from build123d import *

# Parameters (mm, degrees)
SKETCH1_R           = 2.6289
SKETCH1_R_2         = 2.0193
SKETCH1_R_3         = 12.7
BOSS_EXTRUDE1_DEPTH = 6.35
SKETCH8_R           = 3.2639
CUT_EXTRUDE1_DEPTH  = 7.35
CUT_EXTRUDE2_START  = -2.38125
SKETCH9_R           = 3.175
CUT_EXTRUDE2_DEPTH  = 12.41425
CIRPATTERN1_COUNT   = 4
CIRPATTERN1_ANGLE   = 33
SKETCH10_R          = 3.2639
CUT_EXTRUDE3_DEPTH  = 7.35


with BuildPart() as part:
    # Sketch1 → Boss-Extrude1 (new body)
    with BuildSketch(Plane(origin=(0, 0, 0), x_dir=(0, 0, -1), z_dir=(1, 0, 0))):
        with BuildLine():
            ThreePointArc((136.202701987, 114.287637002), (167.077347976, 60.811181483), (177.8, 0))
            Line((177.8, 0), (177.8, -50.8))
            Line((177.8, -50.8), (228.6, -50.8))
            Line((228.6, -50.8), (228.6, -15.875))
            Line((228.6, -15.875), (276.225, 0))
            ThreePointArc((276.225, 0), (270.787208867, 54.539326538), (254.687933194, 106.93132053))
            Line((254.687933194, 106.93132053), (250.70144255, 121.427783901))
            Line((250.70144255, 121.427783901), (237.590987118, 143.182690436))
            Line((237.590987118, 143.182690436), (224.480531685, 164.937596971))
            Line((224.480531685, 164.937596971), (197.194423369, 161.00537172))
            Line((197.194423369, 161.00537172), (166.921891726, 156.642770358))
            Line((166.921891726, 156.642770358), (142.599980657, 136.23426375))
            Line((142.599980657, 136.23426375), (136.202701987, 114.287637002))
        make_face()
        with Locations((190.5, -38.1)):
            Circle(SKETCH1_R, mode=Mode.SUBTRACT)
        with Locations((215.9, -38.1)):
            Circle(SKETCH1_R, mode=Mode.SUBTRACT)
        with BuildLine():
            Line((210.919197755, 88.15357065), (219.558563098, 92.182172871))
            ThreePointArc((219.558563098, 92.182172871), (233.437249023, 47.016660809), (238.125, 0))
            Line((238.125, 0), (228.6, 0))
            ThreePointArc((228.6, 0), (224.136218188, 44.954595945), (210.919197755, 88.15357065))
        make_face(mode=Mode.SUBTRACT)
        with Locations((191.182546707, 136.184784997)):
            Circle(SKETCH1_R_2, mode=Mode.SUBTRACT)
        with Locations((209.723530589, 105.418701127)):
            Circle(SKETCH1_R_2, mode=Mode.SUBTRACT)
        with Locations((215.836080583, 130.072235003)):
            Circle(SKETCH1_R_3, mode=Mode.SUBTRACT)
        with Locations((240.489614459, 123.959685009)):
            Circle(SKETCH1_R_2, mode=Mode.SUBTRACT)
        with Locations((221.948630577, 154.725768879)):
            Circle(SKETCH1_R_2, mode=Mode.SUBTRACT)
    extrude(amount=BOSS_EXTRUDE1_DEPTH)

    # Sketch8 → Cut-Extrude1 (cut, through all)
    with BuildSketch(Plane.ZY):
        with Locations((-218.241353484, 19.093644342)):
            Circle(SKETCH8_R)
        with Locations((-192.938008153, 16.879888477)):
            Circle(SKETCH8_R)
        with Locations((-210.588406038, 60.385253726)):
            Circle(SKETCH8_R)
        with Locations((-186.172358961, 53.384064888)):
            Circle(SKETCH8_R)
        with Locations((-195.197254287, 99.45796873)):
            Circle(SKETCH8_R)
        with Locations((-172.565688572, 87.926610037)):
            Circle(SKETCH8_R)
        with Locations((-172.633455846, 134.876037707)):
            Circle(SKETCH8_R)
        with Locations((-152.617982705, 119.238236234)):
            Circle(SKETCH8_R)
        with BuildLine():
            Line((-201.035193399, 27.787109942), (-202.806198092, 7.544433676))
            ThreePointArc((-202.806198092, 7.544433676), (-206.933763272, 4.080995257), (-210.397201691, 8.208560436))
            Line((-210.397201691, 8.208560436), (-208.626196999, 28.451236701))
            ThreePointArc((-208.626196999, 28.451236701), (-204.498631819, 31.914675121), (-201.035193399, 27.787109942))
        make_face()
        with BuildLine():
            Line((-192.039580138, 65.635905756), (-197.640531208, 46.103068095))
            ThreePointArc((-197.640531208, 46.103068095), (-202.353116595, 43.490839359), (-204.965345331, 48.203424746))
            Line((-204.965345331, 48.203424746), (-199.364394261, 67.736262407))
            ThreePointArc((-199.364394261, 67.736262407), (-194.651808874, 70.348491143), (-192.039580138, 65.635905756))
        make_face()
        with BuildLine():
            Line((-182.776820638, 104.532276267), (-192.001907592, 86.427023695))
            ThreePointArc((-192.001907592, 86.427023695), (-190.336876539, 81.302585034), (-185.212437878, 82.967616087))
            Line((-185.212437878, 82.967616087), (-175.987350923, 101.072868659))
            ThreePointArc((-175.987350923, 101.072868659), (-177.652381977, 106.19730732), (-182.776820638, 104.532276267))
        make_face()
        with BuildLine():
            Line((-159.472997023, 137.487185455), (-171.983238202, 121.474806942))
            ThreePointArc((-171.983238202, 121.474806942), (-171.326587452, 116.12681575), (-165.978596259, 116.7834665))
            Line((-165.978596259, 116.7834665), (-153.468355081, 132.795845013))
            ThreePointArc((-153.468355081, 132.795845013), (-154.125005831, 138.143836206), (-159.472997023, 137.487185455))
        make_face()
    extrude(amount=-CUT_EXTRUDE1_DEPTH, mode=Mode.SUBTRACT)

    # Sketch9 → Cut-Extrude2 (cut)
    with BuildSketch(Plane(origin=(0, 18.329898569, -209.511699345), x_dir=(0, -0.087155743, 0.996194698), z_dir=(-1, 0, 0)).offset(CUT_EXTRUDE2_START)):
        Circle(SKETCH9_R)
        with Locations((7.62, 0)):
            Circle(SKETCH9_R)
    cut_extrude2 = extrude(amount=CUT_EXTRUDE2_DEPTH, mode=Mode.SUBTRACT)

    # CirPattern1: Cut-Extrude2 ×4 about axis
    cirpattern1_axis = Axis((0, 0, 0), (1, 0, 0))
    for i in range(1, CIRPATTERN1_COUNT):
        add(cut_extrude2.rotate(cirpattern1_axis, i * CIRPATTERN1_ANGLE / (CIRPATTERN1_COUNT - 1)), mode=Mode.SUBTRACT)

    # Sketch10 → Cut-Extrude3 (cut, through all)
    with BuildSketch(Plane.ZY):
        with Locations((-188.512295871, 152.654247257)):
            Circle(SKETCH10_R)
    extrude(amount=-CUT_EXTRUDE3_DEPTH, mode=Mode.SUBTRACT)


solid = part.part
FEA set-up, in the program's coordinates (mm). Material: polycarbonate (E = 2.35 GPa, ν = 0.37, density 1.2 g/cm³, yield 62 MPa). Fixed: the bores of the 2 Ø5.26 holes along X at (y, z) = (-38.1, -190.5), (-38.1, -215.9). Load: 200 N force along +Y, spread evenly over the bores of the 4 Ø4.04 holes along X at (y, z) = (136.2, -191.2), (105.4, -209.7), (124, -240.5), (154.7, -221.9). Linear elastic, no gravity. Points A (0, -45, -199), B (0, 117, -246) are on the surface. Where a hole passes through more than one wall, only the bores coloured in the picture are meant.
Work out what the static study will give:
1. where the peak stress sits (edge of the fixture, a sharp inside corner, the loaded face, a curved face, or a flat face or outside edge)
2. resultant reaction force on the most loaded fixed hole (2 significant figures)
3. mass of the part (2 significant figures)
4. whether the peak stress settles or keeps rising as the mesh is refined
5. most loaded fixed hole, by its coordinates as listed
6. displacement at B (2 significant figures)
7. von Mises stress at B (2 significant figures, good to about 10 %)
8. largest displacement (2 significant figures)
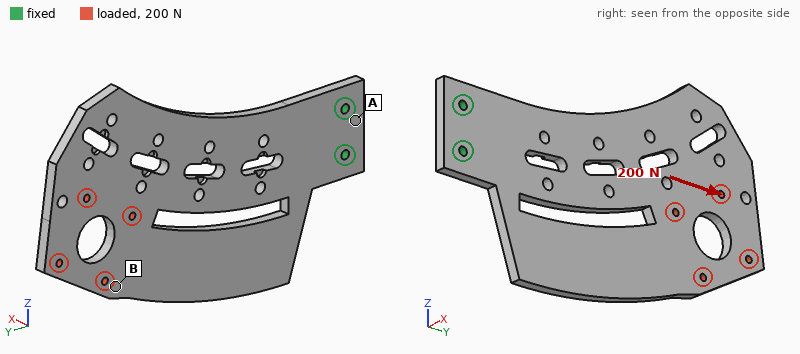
edge of the fixture
190 N
130 g
keeps rising
(-38.1, -215.9)
0.15 mm
0.73 MPa
0.19 mm
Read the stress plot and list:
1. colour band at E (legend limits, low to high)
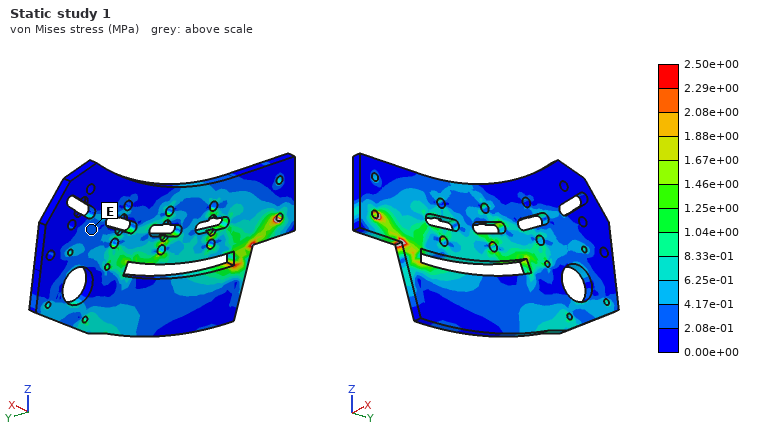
2.08e-01 to 4.17e-01 MPa
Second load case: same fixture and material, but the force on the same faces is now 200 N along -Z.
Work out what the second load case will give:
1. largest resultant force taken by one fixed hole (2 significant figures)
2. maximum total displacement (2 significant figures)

1.2 kN
2.7 mm
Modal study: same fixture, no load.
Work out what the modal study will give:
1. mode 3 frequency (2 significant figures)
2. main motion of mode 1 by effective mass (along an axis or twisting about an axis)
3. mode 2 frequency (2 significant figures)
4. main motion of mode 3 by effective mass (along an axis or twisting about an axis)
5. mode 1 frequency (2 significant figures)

200 Hz
along X
98 Hz
along Z
30 Hz
